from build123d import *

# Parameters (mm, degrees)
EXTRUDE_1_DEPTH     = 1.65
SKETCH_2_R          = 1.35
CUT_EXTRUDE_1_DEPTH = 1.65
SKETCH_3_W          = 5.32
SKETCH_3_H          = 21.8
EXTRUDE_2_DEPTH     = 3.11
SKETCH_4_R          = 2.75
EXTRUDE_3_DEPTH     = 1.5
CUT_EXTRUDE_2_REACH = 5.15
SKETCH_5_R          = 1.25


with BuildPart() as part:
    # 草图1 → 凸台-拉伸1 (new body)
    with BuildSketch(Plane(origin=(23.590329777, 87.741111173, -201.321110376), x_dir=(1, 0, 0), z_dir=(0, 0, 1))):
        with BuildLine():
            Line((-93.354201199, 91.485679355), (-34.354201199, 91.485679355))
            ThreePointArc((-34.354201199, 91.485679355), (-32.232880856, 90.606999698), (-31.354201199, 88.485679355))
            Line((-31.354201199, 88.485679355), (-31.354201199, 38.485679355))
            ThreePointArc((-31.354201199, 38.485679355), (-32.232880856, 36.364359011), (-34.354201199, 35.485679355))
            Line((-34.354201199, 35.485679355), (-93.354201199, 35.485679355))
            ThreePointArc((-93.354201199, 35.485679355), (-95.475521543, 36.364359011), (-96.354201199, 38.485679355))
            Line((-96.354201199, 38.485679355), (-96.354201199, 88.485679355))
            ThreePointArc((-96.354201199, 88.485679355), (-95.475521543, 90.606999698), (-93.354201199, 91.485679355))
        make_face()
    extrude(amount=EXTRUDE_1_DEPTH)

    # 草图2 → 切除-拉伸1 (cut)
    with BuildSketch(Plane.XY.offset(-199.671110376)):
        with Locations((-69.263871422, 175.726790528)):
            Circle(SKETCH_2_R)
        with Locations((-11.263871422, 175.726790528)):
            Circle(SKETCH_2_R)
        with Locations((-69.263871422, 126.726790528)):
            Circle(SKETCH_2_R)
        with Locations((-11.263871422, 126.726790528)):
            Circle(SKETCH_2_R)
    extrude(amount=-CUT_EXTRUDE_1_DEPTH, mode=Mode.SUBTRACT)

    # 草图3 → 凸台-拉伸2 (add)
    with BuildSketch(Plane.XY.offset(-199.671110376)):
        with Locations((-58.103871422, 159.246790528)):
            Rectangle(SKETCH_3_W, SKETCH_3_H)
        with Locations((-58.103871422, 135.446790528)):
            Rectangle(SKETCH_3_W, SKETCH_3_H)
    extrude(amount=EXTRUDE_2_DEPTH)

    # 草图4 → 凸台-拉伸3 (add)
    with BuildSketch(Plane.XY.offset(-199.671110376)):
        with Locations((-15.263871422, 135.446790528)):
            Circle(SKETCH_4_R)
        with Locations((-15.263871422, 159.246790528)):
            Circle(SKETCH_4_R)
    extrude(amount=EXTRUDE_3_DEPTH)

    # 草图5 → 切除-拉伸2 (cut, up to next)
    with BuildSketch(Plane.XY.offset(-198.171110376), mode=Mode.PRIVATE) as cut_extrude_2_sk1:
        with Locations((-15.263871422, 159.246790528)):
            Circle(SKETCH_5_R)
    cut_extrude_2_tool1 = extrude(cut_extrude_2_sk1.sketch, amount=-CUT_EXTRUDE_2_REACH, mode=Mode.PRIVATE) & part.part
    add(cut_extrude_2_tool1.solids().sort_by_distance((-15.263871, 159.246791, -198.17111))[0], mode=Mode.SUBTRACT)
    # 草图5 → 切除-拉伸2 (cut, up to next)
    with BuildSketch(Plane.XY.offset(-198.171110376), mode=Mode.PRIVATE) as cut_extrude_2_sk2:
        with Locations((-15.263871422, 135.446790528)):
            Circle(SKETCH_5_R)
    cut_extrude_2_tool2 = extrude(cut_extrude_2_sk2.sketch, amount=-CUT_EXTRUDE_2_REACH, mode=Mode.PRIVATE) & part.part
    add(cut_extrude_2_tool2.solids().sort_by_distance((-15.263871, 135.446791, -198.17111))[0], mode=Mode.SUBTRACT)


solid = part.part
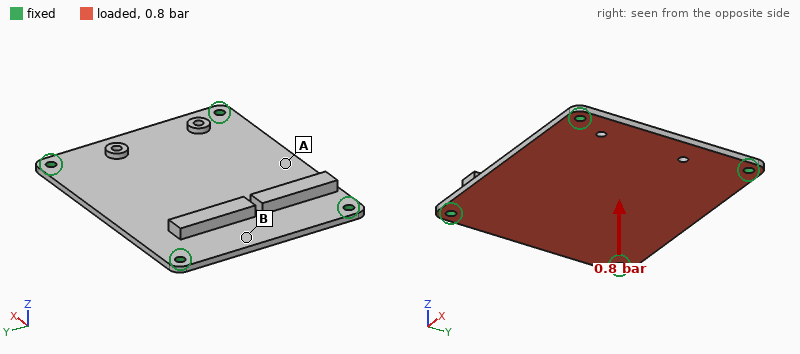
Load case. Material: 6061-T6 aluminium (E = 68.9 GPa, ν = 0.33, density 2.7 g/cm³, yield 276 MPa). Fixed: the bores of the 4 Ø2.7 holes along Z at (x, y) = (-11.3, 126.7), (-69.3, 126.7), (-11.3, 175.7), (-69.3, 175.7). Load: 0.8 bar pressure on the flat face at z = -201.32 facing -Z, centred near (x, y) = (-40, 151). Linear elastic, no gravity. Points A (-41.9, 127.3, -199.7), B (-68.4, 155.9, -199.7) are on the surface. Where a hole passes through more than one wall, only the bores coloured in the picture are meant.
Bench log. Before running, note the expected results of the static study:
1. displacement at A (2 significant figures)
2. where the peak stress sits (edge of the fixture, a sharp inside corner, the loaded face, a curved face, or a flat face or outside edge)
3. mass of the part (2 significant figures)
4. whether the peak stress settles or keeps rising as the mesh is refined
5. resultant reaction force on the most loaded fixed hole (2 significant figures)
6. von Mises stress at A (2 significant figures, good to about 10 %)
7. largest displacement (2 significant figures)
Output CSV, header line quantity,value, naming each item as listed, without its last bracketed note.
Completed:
quantity,value
displacement at A,0.13 mm
where the peak stress sits,edge of the fixture
mass of the part,18 g
whether the peak stress settles or keeps rising as the mesh is refined,keeps rising
resultant reaction force on the most loaded fixed hole,75 N
von Mises stress at A,32 MPa
largest displacement,0.17 mm
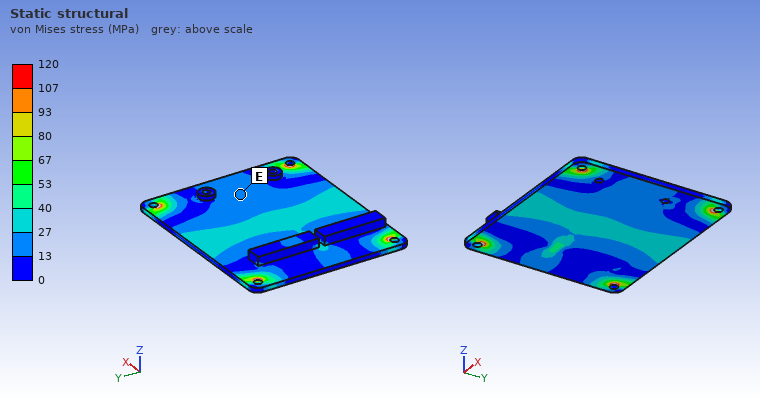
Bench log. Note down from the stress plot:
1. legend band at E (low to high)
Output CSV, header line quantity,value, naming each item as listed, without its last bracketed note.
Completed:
quantity,value
legend band at E,13 to 27 MPa
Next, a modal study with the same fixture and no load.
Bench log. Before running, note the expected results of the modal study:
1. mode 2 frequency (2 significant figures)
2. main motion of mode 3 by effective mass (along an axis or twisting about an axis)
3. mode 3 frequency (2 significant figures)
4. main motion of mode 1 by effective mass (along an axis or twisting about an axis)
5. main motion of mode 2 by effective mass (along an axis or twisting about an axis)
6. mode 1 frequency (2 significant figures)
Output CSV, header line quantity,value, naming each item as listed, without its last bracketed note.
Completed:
quantity,value
mode 2 frequency,3400 Hz
main motion of mode 3 by effective mass,twisting about Y
mode 3 frequency,3700 Hz
main motion of mode 1 by effective mass,along Z
main motion of mode 2 by effective mass,twisting about X
mode 1 frequency,1900 Hz
